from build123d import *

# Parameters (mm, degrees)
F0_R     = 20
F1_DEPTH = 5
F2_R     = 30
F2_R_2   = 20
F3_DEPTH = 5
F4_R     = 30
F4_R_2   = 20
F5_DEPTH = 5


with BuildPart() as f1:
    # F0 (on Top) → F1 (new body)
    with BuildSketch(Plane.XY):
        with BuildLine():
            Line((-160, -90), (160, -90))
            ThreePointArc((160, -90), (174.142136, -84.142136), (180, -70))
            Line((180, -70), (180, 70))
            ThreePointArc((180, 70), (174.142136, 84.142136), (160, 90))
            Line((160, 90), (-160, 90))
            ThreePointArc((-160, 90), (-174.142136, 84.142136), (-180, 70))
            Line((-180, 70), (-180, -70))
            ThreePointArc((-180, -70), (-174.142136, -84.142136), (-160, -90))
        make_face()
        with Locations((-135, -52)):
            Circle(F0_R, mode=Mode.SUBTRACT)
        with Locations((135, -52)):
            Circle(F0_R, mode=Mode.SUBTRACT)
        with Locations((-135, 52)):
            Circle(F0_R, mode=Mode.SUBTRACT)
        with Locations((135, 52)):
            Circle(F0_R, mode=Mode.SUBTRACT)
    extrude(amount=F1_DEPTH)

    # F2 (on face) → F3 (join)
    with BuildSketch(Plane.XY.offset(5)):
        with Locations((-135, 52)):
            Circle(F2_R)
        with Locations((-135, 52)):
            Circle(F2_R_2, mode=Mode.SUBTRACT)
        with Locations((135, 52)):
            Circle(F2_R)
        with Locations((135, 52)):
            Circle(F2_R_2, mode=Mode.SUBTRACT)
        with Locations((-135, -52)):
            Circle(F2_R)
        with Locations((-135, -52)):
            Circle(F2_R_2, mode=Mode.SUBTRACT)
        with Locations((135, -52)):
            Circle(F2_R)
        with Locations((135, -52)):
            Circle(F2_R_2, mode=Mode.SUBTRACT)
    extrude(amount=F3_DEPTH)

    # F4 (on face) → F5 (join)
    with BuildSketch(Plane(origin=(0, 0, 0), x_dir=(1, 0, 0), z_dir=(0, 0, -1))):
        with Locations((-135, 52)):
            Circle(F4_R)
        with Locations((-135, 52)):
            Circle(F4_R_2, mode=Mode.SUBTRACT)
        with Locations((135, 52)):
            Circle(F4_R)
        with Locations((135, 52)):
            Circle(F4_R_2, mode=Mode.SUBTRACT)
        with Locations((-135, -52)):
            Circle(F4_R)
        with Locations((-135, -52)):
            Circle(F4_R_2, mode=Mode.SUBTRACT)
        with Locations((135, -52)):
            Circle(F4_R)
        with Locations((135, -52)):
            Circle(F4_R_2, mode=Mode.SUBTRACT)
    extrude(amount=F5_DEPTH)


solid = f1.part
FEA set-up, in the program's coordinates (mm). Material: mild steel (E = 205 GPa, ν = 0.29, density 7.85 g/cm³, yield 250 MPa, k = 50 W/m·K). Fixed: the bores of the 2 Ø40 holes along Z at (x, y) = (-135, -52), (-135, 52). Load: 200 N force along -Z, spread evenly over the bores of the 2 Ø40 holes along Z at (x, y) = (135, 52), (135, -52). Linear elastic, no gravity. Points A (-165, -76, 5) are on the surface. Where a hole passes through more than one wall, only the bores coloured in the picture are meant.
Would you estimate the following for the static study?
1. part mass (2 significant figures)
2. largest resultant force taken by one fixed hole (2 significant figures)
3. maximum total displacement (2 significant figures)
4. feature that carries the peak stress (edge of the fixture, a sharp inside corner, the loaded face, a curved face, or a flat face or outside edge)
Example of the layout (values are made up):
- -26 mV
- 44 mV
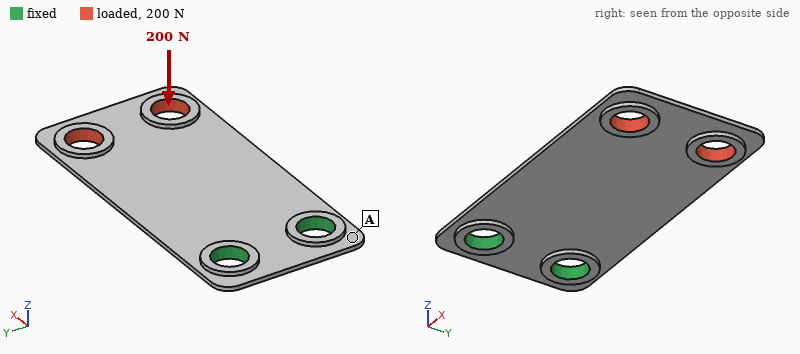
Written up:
- 2.8 kg
- 100 N
- 3.1 mm
- a flat face or outside edge
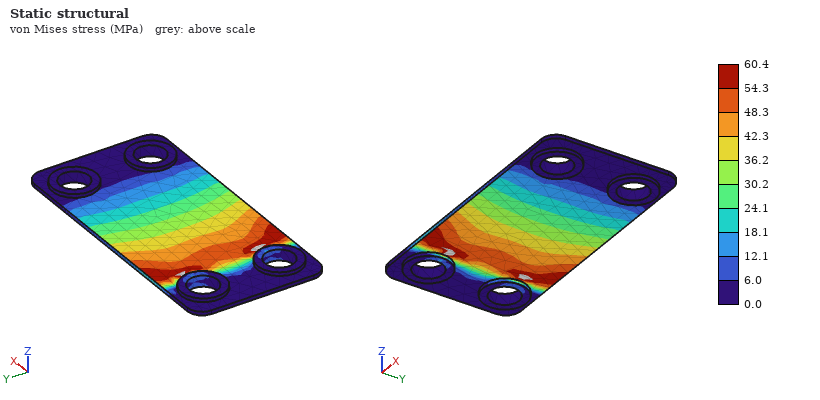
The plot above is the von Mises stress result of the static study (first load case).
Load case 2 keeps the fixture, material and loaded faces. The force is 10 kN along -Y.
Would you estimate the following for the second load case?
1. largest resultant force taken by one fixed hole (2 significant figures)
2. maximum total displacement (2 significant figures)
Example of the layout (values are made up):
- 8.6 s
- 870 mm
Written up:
- 21 kN
- 0.19 mm
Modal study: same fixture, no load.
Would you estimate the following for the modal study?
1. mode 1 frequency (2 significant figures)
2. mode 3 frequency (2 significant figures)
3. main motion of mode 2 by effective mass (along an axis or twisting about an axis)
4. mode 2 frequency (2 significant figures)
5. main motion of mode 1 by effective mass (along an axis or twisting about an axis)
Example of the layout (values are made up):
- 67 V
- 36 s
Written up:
- 46 Hz
- 310 Hz
- twisting about X
- 170 Hz
- along Z
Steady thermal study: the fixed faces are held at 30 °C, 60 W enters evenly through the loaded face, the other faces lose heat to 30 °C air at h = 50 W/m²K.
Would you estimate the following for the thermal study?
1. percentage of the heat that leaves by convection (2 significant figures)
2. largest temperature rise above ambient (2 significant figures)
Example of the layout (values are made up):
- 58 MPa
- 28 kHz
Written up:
- 99 %
- 36 K
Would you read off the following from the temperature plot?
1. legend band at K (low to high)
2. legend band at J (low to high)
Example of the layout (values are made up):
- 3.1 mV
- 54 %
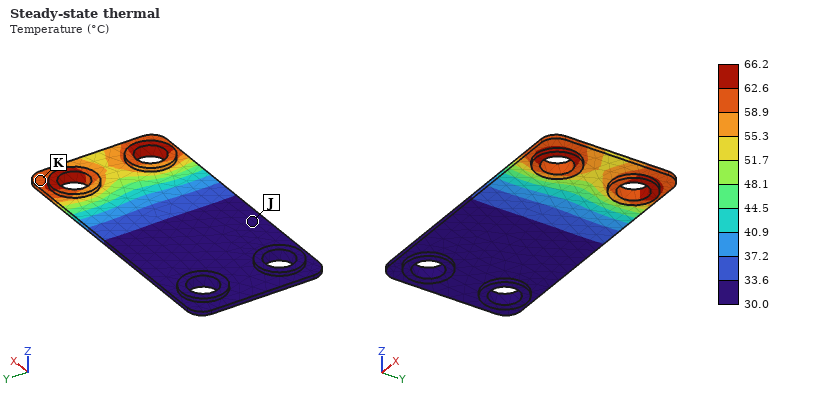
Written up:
- 58.9 to 62.6 °C
- 30.0 to 33.6 °C
